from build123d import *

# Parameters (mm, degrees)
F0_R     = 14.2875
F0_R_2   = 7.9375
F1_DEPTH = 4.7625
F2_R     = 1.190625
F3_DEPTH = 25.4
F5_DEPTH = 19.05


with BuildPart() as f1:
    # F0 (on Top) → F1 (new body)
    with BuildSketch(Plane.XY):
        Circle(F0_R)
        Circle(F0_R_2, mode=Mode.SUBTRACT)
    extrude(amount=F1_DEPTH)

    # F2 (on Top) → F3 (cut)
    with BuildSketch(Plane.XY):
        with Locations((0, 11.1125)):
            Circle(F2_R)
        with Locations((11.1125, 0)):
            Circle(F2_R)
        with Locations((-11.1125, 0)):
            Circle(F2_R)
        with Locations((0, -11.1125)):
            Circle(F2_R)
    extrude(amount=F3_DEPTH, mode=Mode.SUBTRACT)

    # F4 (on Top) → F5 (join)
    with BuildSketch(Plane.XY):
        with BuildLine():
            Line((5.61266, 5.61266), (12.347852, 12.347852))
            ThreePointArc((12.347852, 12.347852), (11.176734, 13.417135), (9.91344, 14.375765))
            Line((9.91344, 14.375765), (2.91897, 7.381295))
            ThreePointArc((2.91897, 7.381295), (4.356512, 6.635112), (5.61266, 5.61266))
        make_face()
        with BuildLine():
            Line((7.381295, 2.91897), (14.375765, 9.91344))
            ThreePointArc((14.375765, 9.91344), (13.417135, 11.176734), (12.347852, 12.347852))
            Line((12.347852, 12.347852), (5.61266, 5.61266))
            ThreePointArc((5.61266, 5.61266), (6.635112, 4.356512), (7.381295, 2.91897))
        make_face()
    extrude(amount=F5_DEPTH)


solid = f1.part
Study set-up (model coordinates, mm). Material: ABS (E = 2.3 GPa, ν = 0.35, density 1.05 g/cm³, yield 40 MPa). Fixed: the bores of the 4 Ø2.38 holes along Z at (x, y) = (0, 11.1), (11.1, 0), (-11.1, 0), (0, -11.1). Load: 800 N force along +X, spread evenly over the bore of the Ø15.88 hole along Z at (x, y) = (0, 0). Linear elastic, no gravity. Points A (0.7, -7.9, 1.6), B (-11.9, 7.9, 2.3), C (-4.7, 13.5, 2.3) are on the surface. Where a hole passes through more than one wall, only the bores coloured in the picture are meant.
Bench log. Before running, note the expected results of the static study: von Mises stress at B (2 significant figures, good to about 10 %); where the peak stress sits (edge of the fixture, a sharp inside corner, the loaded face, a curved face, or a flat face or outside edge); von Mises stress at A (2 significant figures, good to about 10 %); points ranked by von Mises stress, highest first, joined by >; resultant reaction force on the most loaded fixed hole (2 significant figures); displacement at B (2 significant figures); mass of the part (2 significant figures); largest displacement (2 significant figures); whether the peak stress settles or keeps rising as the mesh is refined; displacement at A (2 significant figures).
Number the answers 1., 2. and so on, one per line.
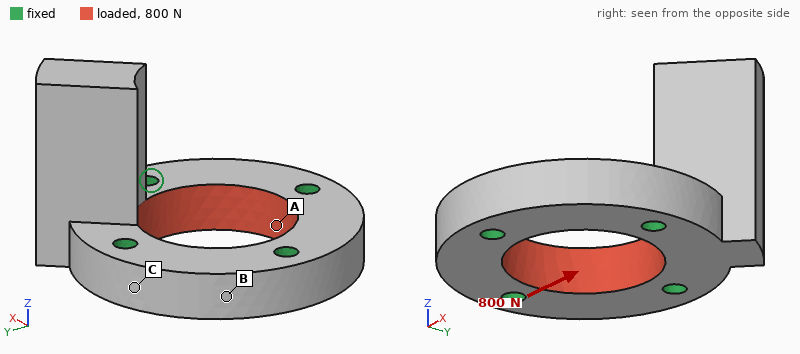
1. 3.4 MPa
2. edge of the fixture
3. 5.9 MPa
4. A > B > C
5. 230 N
6. 16 µm
7. 3.1 g
8. 23 µm
9. keeps rising
10. 16 µm
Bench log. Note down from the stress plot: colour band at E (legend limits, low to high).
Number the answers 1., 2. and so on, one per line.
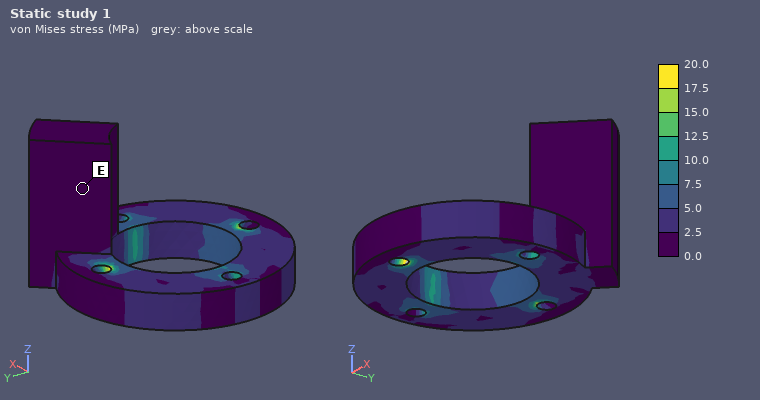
1. 0.0 to 2.5 MPa
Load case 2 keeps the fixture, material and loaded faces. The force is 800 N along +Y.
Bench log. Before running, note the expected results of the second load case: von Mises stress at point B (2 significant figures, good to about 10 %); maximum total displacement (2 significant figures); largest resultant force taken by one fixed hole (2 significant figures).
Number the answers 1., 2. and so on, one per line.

1. 3.2 MPa
2. 23 µm
3. 230 N
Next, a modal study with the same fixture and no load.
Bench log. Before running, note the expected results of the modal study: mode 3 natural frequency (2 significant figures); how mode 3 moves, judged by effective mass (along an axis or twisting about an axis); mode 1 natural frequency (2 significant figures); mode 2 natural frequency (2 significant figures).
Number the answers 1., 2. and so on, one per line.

1. 9300 Hz
2. along Z
3. 2600 Hz
4. 4300 Hz
